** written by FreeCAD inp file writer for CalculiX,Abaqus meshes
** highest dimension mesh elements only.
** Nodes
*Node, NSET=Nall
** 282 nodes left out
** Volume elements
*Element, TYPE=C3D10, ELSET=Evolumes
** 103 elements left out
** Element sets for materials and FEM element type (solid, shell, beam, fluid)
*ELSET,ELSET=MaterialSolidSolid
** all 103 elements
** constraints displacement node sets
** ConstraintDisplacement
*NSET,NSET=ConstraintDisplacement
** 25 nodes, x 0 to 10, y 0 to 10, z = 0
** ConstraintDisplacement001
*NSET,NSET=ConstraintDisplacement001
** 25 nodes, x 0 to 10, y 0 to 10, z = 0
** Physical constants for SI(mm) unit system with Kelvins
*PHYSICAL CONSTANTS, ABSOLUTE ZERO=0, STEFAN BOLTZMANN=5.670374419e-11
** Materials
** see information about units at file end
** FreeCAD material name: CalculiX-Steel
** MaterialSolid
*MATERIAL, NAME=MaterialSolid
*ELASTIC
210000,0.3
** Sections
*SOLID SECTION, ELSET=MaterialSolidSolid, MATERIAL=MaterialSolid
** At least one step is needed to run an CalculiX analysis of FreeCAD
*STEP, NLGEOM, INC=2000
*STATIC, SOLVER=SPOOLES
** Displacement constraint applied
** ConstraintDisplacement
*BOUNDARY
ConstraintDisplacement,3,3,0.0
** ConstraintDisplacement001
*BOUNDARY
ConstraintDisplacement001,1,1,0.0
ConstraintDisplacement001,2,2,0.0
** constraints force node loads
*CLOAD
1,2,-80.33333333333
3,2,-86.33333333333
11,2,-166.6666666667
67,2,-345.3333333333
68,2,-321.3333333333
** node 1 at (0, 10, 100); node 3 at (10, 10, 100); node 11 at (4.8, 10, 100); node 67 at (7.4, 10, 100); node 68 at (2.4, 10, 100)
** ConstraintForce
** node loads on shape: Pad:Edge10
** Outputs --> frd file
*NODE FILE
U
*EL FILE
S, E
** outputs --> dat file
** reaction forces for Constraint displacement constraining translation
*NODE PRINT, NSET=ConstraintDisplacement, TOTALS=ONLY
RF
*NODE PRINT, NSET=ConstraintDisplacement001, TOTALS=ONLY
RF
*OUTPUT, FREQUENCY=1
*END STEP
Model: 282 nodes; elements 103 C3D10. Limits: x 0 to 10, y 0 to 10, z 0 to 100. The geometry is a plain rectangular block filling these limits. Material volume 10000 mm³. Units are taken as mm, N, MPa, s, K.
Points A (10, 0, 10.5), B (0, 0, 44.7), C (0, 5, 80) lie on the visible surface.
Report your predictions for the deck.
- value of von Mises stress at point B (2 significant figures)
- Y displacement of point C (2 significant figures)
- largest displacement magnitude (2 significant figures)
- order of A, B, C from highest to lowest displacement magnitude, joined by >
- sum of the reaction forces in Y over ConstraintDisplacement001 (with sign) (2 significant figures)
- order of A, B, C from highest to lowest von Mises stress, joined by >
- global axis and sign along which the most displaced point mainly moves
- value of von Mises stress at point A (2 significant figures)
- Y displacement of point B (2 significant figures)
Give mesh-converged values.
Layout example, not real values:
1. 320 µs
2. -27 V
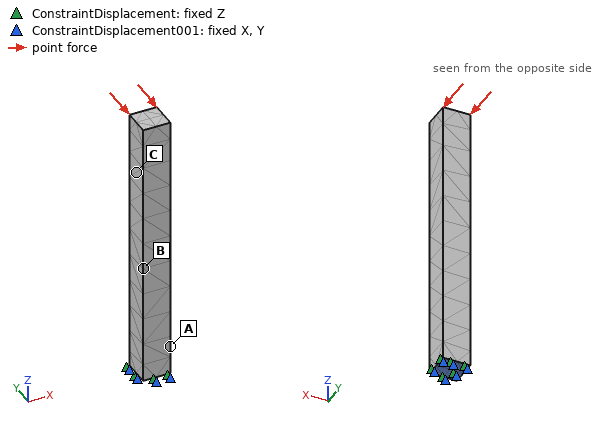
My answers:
1. 330 MPa
2. -1.3 mm
3. 1.9 mm
4. C > B > A
5. 1000 N
6. A > B > C
7. -Y
8. 540 MPa
9. -0.48 mm
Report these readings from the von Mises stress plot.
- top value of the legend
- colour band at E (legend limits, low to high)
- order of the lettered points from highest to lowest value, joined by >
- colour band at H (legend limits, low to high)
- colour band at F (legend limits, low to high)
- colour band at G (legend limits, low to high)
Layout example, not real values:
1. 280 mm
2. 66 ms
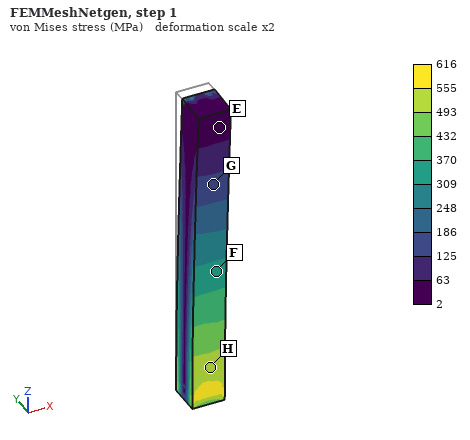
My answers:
1. 616 MPa
2. 2 to 63 MPa
3. H > F > G > E
4. 493 to 555 MPa
5. 309 to 370 MPa
6. 125 to 186 MPa
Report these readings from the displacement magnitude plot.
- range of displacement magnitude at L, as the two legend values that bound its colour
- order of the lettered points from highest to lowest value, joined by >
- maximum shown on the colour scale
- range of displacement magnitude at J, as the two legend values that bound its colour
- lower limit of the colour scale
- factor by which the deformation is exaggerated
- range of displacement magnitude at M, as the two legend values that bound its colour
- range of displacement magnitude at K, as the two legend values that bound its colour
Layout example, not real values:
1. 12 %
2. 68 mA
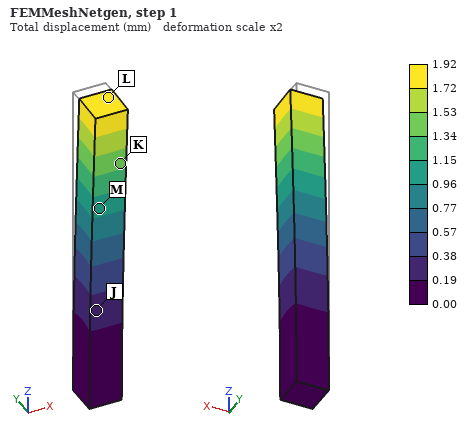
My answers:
1. 1.72 to 1.92 mm
2. L > K > M > J
3. 1.92 mm
4. 0.19 to 0.38 mm
5. 0.00 mm
6. 2
7. 0.96 to 1.15 mm
8. 1.34 to 1.53 mm
